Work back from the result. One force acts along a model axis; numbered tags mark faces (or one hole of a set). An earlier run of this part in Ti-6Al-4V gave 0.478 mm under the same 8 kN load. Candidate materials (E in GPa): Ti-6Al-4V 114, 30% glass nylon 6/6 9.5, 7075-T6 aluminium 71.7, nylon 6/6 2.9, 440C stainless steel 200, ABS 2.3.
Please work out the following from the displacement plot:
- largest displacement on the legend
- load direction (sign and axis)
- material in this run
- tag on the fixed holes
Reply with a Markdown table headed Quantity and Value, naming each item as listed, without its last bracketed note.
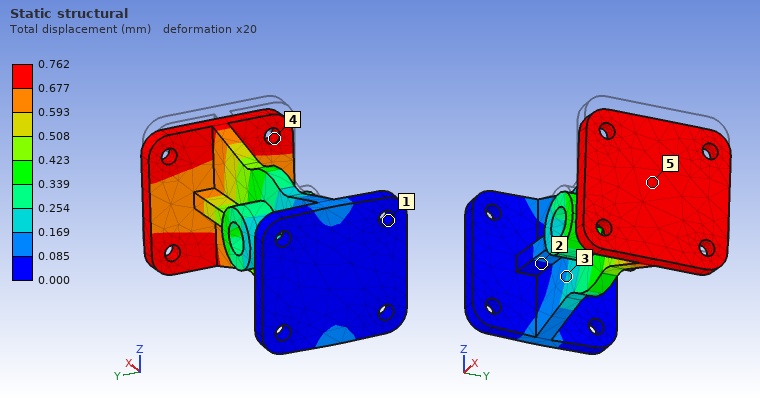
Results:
| Quantity | Value |
|---|---|
| largest displacement on the legend | 0.762 mm |
| load direction | -Z |
| material in this run | 7075-T6 aluminium |
| tag on the fixed holes | 1 |
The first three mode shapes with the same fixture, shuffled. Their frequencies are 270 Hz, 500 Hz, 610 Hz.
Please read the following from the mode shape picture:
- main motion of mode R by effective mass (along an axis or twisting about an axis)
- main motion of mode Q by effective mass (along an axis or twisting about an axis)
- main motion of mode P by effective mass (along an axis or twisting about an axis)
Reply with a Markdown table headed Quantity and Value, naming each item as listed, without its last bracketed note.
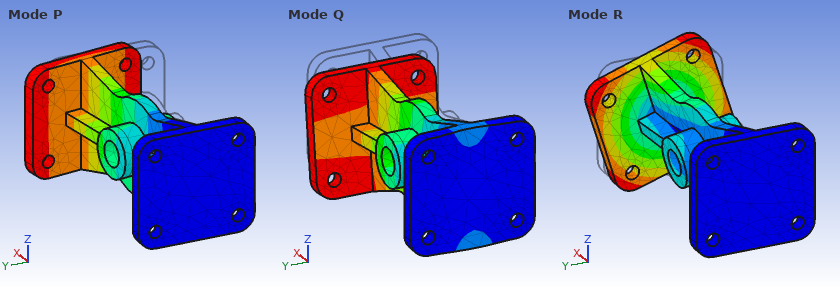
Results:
| Quantity | Value |
|---|---|
| main motion of mode R by effective mass | twisting about X |
| main motion of mode Q by effective mass | along Z |
| main motion of mode P by effective mass | along Y |
